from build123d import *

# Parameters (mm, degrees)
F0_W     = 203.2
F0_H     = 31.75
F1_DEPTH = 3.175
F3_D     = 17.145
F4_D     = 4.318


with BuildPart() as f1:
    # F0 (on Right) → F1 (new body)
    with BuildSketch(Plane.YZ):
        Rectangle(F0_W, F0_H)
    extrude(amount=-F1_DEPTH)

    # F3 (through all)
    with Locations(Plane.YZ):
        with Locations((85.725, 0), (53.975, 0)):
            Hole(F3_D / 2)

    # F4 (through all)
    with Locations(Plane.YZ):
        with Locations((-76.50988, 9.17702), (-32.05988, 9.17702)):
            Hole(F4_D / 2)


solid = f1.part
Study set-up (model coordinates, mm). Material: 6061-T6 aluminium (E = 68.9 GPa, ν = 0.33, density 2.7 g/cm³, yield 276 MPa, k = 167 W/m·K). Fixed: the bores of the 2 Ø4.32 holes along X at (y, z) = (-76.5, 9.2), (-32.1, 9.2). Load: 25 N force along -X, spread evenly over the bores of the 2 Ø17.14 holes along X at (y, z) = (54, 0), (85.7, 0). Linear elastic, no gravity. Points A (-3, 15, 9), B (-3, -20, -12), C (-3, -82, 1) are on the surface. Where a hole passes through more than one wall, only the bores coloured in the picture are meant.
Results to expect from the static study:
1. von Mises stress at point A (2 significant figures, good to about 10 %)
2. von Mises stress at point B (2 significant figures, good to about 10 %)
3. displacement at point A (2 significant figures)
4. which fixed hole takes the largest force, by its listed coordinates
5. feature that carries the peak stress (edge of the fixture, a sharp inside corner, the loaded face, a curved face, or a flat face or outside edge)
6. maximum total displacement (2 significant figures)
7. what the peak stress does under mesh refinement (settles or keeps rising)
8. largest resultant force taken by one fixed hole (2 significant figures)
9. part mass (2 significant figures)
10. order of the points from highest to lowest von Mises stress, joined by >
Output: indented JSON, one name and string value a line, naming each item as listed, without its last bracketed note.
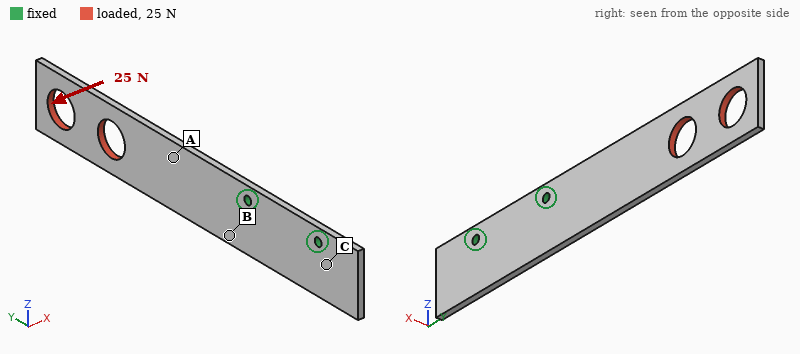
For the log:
{
  "von Mises stress at point A": "26 MPa",
  "von Mises stress at point B": "36 MPa",
  "displacement at point A": "0.44 mm",
  "which fixed hole takes the largest force, by its listed coordinates": "(-32.1, 9.2)",
  "feature that carries the peak stress": "edge of the fixture",
  "maximum total displacement": "2.4 mm",
  "what the peak stress does under mesh refinement": "keeps rising",
  "largest resultant force taken by one fixed hole": "43 N",
  "part mass": "51 g",
  "order of the points from highest to lowest von Mises stress, joined by >": "B > A > C"
}
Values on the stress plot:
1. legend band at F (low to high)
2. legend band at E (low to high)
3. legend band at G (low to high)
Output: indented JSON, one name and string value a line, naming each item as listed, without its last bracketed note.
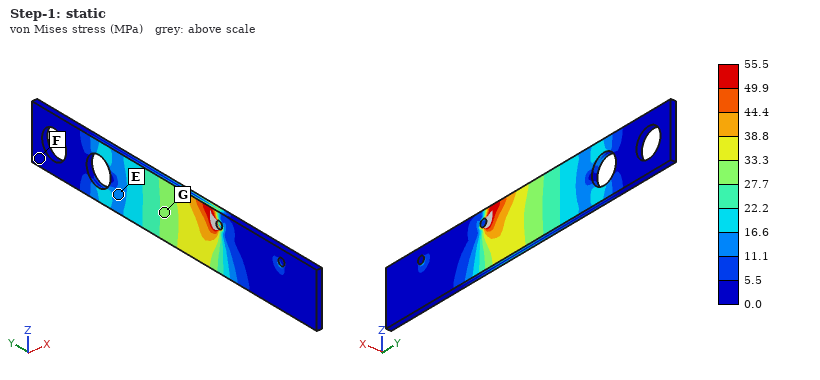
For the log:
{
  "legend band at F": "0.0 to 5.5 MPa",
  "legend band at E": "11.1 to 16.6 MPa",
  "legend band at G": "27.7 to 33.3 MPa"
}
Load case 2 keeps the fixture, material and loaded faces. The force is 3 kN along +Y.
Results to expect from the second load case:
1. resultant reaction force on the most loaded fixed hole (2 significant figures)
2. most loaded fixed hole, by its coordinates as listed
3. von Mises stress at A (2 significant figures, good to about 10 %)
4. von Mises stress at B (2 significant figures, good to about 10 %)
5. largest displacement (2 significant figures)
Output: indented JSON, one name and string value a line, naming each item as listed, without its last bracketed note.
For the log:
{
  "resultant reaction force on the most loaded fixed hole": "2.3 kN",
  "most loaded fixed hole, by its coordinates as listed": "(-32.1, 9.2)",
  "von Mises stress at A": "30 MPa",
  "von Mises stress at B": "30 MPa",
  "largest displacement": "0.12 mm"
}
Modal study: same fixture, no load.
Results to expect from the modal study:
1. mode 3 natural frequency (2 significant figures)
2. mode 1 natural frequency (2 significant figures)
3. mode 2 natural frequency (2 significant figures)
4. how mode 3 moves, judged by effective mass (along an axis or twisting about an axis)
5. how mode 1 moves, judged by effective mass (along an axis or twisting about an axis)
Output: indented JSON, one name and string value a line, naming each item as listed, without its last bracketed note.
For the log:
{
  "mode 3 natural frequency": "1100 Hz",
  "mode 1 natural frequency": "160 Hz",
  "mode 2 natural frequency": "840 Hz",
  "how mode 3 moves, judged by effective mass": "twisting about Y",
  "how mode 1 moves, judged by effective mass": "along X"
}
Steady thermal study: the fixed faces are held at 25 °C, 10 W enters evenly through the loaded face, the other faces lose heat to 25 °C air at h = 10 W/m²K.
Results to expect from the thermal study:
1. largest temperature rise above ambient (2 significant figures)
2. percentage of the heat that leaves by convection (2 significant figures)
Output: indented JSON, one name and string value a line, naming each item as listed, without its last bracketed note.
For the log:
{
  "largest temperature rise above ambient": "59 K",
  "percentage of the heat that leaves by convection": "28 %"
}
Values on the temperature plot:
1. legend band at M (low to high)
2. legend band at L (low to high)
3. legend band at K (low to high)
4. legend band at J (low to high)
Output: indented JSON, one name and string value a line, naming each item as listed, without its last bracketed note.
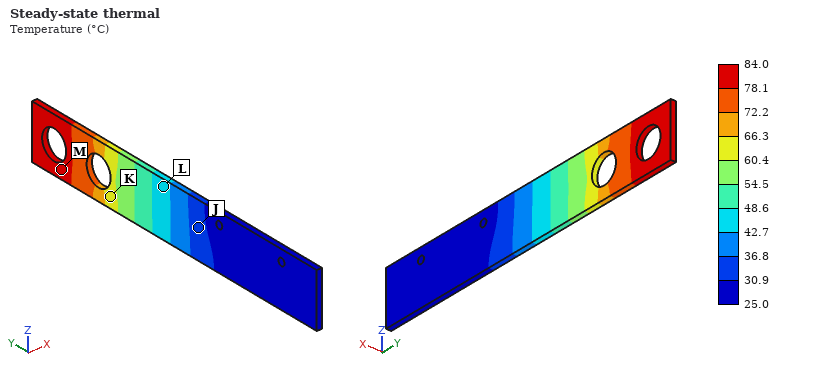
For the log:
{
  "legend band at M": "78.1 to 84.0 °C",
  "legend band at L": "42.7 to 48.6 °C",
  "legend band at K": "60.4 to 66.3 °C",
  "legend band at J": "30.9 to 36.8 °C"
}
